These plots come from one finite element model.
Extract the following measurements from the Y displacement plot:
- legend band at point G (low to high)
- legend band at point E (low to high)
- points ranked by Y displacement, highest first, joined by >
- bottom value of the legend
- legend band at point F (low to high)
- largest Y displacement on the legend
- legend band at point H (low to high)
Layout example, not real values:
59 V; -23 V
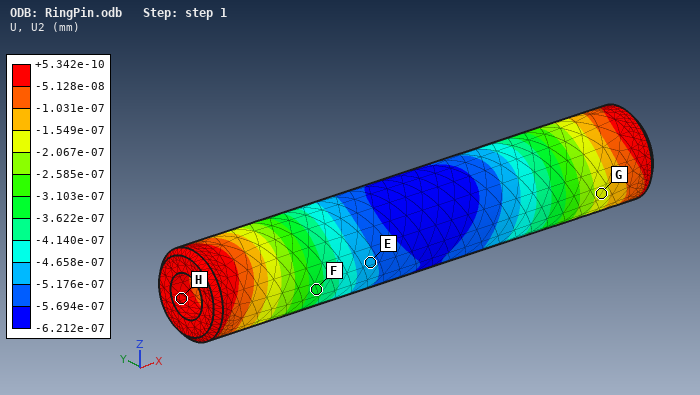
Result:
-2.067e-07 to -1.549e-07 mm; -5.176e-07 to -4.658e-07 mm; H > G > F > E; -6.212e-07 mm; -3.622e-07 to -3.103e-07 mm; +5.342e-10 mm; -5.128e-08 to +5.342e-10 mm
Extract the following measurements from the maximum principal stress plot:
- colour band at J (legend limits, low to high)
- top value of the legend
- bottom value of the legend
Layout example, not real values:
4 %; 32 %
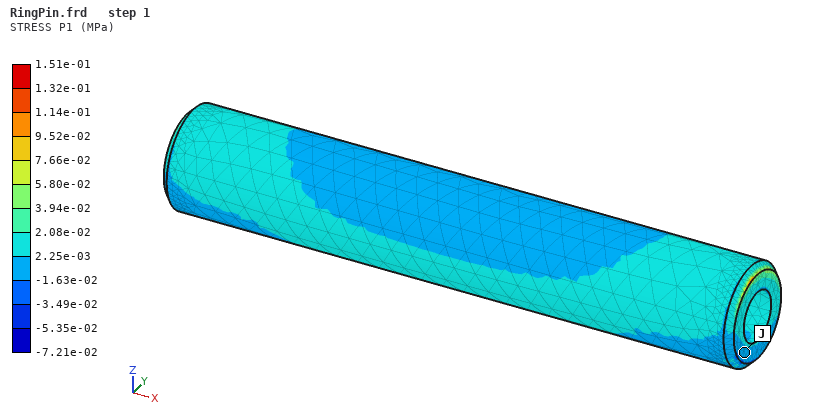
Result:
-1.63e-02 to 2.25e-03 MPa; 1.51e-01 MPa; -7.21e-02 MPa
